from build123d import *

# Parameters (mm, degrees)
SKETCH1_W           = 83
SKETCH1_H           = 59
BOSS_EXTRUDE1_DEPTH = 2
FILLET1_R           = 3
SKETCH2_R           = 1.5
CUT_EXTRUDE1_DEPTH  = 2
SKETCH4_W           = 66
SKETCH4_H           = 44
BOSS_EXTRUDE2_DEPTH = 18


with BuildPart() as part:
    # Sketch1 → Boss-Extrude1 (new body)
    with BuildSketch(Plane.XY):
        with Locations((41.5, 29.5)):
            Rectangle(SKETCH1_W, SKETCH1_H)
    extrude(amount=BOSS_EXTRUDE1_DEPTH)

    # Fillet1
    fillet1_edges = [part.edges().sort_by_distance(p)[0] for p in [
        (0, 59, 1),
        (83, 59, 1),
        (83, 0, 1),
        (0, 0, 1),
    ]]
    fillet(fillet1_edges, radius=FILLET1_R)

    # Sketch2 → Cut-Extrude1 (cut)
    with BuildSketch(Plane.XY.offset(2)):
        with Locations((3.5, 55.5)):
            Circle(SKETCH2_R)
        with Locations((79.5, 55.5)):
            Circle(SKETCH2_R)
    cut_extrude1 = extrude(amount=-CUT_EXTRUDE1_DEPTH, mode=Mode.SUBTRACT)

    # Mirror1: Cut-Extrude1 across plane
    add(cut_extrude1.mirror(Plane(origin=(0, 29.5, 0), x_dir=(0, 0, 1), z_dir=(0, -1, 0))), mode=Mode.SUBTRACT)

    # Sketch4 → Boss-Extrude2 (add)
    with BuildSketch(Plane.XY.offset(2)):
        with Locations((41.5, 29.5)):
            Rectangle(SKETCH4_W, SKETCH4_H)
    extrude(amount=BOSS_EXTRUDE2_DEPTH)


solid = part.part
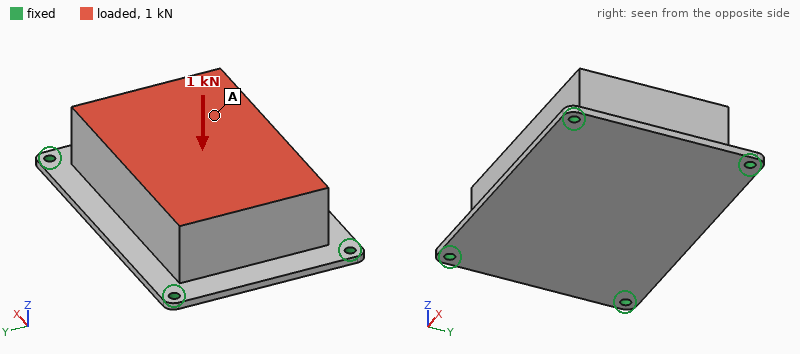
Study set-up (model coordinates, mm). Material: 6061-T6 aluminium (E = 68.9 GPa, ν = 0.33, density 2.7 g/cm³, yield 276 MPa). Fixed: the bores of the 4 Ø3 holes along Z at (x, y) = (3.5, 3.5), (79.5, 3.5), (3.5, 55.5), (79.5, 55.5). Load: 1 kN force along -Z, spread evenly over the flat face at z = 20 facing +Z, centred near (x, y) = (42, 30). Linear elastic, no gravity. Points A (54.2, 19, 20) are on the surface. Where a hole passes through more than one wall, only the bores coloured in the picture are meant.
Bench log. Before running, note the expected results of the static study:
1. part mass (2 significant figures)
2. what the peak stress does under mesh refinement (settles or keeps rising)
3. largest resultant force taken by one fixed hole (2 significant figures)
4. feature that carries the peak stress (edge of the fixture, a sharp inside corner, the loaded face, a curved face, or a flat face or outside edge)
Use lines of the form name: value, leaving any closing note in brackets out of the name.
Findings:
part mass: 170 g
what the peak stress does under mesh refinement: keeps rising
largest resultant force taken by one fixed hole: 290 N
feature that carries the peak stress: edge of the fixture
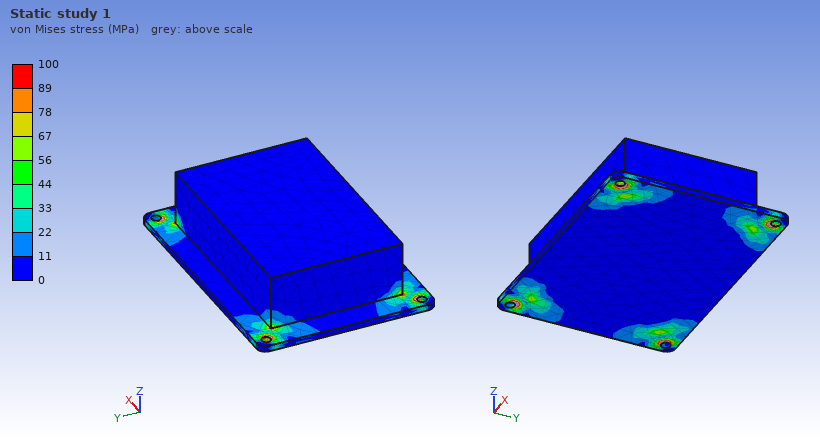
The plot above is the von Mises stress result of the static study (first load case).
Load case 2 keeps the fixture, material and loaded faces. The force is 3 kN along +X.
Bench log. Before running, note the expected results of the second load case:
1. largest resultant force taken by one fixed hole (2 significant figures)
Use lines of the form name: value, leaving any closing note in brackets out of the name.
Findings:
largest resultant force taken by one fixed hole: 920 N
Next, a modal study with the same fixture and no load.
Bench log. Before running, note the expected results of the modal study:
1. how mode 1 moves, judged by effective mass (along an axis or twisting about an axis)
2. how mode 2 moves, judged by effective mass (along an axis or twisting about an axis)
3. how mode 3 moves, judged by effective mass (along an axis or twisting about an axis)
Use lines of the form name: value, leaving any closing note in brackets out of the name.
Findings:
how mode 1 moves, judged by effective mass: along Z
how mode 2 moves, judged by effective mass: along Y
how mode 3 moves, judged by effective mass: along X
